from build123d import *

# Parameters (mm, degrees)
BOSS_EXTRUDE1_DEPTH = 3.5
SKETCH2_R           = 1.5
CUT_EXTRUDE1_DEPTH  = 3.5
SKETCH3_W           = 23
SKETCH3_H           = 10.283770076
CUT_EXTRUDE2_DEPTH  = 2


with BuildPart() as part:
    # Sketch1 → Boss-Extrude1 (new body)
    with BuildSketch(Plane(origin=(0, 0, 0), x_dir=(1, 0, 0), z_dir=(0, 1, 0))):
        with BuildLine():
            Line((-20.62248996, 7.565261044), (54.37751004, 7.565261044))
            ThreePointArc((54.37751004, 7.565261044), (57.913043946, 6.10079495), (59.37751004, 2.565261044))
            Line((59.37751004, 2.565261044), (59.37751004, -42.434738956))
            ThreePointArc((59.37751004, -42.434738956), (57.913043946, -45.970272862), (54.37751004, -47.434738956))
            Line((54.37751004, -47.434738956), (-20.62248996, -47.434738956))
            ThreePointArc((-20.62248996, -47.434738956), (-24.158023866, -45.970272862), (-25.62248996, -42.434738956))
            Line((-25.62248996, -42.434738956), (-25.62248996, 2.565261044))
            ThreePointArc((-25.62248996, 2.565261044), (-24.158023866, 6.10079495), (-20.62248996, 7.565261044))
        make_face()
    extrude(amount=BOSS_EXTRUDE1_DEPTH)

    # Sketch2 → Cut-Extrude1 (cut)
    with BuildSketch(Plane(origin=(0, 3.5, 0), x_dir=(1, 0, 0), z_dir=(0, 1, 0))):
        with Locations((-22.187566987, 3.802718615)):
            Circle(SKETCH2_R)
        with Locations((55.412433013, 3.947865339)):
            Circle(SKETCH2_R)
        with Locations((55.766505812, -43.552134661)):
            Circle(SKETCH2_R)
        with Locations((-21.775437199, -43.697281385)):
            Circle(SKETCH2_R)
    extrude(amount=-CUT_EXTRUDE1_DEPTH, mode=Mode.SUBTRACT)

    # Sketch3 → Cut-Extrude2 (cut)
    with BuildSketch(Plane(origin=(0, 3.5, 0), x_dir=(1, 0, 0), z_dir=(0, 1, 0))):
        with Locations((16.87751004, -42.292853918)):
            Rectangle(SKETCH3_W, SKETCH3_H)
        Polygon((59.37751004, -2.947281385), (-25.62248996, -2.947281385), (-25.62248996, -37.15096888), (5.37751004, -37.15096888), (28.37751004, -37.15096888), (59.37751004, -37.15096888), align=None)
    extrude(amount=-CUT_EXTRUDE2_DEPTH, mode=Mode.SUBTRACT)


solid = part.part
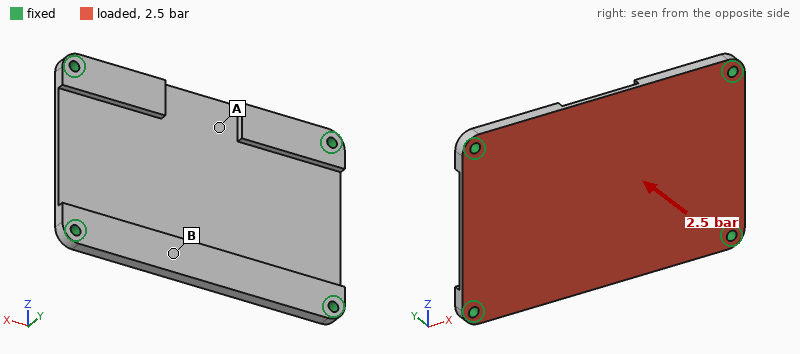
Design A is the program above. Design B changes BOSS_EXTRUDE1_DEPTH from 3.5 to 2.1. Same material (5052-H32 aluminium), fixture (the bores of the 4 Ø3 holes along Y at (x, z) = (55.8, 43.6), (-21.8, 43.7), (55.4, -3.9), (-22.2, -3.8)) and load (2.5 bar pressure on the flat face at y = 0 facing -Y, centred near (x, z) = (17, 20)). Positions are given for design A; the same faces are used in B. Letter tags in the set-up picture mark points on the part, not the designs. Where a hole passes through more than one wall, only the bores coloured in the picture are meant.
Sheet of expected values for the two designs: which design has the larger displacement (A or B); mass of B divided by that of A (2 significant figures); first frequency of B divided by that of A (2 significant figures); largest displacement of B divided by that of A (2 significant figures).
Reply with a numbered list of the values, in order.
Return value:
1. B
2. 0.79
3. 0.61
4. 2.7
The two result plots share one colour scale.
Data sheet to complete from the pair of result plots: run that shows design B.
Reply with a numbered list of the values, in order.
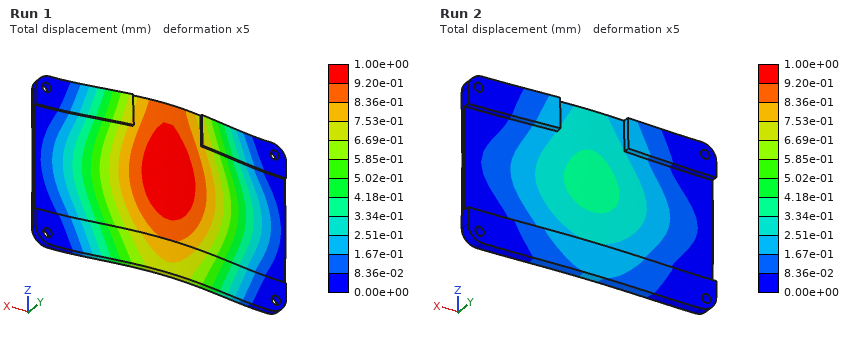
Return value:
1. Run 1
